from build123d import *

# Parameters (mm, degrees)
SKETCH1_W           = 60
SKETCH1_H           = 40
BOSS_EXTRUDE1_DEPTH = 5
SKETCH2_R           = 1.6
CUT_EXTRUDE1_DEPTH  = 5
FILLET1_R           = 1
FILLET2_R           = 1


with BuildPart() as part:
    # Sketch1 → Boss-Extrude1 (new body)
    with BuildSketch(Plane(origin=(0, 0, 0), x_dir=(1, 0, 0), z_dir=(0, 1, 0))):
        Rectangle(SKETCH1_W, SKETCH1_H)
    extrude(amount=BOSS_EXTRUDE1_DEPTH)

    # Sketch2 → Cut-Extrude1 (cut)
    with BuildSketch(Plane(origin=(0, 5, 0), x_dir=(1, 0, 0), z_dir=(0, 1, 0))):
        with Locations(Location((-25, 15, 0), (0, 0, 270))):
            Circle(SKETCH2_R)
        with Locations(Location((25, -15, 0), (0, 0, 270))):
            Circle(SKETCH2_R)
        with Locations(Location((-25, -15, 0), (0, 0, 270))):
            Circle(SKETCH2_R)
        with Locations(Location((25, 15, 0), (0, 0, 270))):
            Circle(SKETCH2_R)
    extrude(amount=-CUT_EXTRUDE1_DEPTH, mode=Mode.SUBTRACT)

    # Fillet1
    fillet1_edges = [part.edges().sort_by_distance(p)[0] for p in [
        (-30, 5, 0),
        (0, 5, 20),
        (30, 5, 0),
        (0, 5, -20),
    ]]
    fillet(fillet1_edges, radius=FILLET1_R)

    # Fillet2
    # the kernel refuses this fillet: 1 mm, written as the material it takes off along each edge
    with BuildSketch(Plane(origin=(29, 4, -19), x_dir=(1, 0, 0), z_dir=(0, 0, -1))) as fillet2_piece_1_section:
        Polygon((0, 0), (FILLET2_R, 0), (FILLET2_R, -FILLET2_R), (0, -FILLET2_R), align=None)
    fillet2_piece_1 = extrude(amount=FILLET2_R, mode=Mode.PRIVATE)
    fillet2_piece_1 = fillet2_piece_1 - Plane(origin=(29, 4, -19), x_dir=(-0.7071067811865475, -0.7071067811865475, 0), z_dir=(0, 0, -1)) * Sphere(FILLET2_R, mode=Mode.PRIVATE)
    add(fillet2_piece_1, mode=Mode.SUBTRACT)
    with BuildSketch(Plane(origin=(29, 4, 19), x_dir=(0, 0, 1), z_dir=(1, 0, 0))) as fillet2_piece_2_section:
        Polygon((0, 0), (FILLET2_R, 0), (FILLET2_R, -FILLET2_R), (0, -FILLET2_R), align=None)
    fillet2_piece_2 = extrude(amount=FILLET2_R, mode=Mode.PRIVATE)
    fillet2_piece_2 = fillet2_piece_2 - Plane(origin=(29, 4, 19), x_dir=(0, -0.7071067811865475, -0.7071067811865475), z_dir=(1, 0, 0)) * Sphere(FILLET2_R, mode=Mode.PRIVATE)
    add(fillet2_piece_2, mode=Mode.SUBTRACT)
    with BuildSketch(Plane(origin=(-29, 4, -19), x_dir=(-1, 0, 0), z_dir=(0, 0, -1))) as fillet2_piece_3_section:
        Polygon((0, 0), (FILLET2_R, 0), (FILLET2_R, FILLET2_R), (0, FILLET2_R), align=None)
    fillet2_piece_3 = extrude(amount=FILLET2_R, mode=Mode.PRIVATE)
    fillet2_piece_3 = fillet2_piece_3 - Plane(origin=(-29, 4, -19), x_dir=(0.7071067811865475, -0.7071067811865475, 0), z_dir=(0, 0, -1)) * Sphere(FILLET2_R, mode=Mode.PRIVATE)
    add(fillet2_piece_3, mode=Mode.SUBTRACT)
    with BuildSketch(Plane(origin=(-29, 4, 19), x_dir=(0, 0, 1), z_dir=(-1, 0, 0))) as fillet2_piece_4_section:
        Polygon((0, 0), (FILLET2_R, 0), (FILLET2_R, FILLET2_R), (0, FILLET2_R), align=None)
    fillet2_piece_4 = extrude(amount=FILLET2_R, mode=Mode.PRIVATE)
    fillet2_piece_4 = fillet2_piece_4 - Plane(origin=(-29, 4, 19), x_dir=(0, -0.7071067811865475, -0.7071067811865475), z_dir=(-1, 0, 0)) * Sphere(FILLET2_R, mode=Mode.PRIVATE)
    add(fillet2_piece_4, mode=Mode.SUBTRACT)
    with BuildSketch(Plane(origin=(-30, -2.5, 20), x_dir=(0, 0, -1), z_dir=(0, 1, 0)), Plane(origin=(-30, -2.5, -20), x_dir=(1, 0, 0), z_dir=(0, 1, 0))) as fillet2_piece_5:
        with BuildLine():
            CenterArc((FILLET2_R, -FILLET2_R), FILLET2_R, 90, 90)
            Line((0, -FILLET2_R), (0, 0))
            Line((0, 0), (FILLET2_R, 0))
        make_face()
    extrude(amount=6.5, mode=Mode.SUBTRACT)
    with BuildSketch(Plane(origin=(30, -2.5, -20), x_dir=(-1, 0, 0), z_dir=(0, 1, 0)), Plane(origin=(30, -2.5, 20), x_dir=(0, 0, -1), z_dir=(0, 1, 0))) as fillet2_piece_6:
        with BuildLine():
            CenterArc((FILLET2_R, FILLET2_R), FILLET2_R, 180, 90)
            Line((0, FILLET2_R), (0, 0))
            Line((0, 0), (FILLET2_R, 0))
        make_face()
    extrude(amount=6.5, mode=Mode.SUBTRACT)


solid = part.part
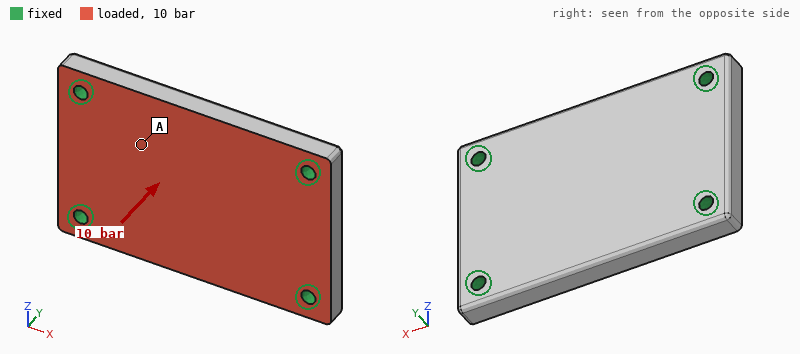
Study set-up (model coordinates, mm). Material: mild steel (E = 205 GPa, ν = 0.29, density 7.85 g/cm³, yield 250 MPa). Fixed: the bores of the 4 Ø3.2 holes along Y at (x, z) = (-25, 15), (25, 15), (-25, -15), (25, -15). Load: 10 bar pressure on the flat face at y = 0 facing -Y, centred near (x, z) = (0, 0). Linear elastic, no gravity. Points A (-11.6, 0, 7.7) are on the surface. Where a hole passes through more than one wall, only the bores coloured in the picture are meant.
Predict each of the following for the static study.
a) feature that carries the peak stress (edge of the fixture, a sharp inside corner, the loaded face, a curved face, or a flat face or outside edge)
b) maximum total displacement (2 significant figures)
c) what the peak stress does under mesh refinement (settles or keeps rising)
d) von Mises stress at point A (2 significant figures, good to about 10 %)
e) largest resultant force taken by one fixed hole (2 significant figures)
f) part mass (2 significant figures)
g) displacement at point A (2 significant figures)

edge of the fixture
11 µm
keeps rising
12 MPa
590 N
93 g
8.0 µm
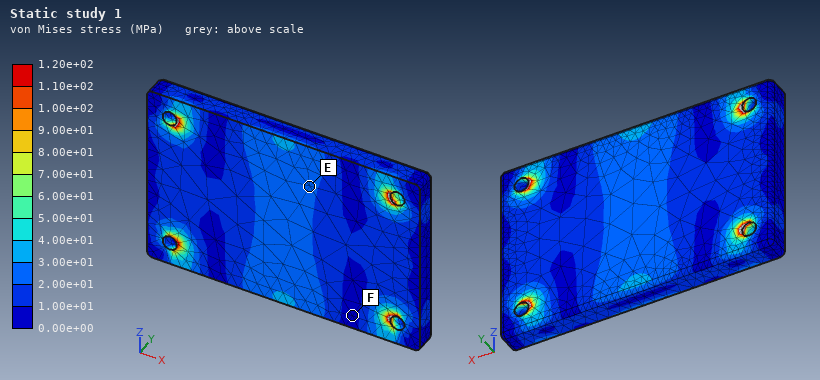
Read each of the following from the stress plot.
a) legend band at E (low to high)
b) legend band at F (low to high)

2.00e+01 to 3.00e+01 MPa
0.00e+00 to 1.00e+01 MPa
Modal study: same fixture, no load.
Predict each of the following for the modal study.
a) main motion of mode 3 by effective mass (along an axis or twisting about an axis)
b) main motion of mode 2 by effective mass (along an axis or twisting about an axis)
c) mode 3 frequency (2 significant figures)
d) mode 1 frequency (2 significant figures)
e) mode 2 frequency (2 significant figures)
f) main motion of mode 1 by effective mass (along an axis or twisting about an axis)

twisting about Z
twisting about X
21 kHz
8600 Hz
13 kHz
along Y
